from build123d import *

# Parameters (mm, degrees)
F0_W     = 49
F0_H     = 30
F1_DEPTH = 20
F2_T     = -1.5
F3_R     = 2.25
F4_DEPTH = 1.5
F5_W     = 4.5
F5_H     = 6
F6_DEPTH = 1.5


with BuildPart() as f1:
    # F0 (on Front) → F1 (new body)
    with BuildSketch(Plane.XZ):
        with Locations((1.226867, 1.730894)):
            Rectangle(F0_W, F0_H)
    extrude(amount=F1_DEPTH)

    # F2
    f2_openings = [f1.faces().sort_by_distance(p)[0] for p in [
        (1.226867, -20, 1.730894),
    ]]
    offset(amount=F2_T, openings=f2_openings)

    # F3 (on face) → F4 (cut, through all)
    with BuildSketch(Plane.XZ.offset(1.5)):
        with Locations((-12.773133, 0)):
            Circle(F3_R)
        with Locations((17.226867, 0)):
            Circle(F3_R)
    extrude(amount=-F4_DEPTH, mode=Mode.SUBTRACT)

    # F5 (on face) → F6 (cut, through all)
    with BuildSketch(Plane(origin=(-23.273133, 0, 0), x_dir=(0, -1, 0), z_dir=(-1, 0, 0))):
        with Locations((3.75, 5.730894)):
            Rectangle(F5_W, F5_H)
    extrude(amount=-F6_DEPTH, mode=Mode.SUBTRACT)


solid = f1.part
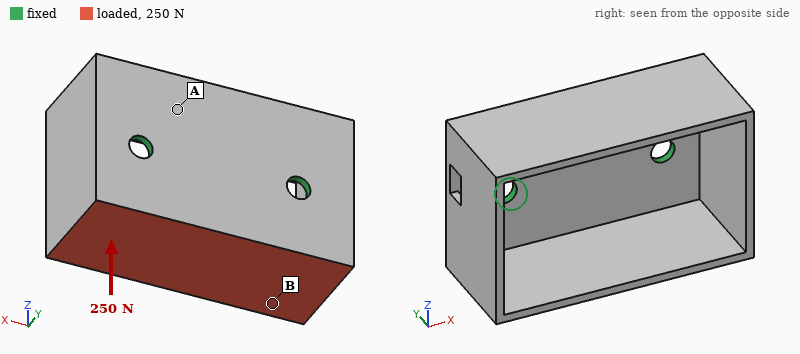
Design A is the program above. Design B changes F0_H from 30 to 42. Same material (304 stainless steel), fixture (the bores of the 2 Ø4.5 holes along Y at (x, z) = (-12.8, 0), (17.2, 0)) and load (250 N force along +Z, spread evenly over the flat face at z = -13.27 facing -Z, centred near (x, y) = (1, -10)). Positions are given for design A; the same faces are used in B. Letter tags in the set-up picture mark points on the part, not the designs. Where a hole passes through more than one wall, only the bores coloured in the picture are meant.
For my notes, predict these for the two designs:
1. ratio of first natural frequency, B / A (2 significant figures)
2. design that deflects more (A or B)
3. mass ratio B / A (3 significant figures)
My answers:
0.72
B
1.24
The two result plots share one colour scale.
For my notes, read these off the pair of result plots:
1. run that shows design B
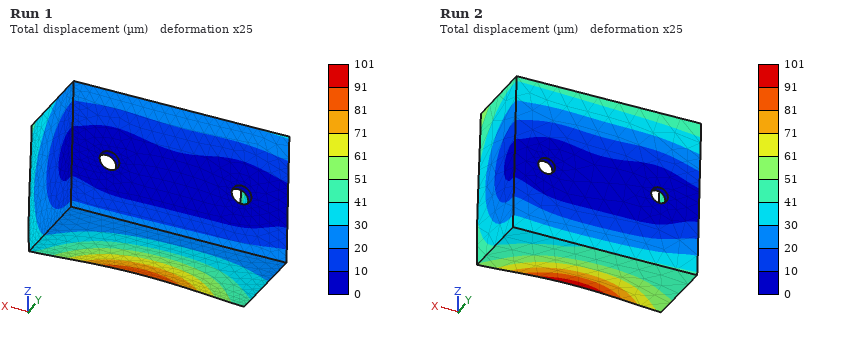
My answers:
Run 2
